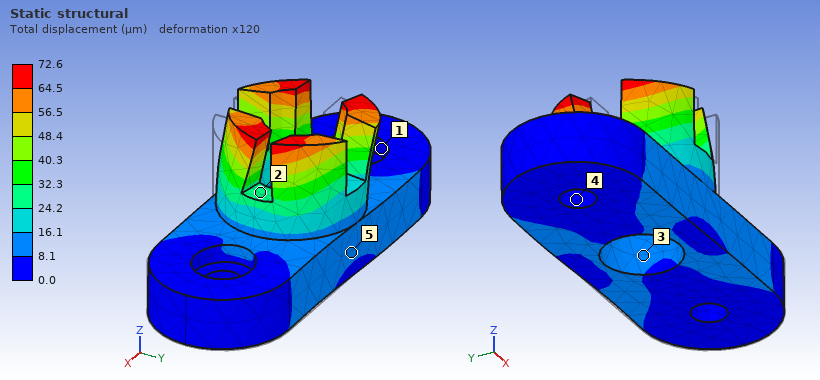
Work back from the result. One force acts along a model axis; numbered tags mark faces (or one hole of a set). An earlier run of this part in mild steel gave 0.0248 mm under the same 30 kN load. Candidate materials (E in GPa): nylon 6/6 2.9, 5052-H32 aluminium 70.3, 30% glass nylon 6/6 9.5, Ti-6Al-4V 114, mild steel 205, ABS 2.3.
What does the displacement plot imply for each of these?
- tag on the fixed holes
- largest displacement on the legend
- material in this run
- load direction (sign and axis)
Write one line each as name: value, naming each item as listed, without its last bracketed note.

tag on the fixed holes: 4
largest displacement on the legend: 72.6 µm
material in this run: 5052-H32 aluminium
load direction: -X
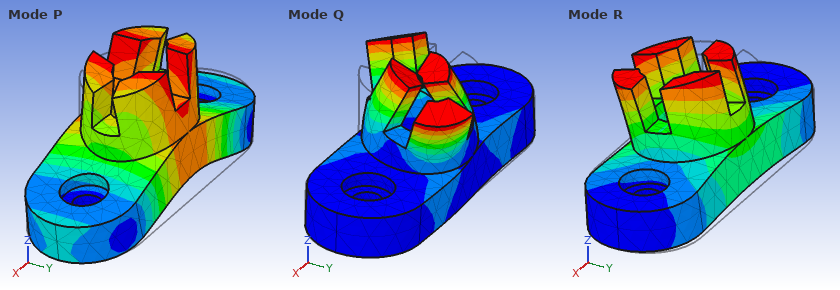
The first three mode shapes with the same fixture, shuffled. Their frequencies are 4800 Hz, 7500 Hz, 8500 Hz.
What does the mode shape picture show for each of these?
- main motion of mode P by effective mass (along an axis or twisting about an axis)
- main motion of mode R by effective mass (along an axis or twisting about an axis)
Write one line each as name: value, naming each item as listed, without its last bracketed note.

main motion of mode P by effective mass: along Z
main motion of mode R by effective mass: along Y
